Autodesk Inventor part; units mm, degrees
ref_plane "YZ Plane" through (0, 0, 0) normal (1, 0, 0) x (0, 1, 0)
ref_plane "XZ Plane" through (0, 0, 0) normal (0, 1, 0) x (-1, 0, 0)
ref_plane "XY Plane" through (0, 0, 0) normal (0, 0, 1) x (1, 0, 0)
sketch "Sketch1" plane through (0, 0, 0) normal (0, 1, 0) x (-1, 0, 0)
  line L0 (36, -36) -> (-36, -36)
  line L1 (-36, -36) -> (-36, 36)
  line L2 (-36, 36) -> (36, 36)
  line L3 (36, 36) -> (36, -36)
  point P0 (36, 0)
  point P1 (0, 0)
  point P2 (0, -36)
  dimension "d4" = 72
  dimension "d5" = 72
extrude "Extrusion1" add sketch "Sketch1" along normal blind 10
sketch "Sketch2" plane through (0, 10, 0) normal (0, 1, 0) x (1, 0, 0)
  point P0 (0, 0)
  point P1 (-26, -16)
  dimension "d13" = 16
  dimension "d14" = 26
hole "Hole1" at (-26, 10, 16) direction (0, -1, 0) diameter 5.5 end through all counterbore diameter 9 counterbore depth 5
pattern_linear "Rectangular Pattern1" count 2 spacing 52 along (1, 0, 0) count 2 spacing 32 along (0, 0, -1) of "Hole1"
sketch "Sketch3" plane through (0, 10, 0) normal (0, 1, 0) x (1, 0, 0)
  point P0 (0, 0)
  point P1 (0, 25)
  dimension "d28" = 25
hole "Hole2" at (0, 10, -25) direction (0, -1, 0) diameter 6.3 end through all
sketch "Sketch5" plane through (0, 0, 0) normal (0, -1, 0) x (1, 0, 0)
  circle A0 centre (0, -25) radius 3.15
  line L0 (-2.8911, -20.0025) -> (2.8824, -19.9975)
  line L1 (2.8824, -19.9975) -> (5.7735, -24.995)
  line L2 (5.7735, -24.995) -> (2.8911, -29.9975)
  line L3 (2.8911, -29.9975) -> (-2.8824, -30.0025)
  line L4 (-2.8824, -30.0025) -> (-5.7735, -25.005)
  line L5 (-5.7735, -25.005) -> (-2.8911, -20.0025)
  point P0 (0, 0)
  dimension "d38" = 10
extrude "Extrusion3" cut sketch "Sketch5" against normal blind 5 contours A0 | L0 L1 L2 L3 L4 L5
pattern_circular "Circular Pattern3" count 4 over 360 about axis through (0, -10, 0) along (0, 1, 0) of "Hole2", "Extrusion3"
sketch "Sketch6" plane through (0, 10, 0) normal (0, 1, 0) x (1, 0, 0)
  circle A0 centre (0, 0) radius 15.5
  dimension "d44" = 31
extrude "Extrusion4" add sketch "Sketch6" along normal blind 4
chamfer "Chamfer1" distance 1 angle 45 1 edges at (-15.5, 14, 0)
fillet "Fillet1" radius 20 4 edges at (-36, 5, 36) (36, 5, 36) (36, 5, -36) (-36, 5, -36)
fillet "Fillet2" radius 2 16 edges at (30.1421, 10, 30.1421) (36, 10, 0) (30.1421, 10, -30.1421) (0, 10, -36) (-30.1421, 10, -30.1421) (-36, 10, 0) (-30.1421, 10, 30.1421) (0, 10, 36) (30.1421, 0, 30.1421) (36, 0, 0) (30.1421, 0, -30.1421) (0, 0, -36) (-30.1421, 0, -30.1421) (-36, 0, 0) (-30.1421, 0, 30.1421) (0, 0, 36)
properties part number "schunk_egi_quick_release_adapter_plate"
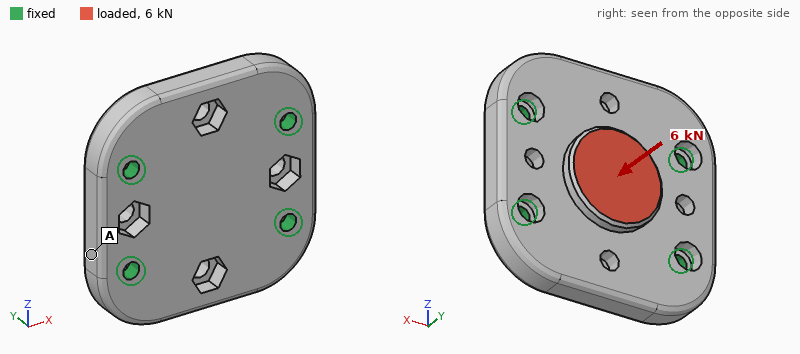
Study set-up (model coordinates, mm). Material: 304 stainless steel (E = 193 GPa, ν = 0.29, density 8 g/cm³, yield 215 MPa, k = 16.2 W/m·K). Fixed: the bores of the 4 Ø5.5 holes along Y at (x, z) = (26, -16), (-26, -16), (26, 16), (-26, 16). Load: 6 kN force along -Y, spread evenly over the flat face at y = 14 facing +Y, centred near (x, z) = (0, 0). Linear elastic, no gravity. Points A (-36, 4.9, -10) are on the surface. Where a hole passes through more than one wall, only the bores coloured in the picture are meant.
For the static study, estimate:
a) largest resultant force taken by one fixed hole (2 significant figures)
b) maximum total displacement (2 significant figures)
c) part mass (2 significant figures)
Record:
2.0 kN
7.6 µm
370 g
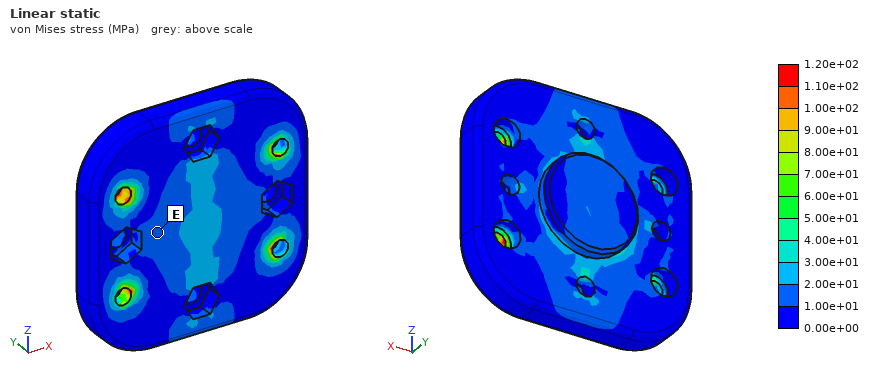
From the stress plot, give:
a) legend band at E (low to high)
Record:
1.00e+01 to 2.00e+01 MPa
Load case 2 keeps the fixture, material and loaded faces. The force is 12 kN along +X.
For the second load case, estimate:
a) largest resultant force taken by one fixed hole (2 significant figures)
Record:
3.5 kN
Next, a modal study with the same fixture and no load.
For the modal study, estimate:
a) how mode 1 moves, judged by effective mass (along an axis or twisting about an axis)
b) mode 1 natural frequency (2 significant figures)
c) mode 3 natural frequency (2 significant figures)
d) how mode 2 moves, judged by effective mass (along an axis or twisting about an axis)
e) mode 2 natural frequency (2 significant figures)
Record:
twisting about X
9500 Hz
15 kHz
along Y
9900 Hz
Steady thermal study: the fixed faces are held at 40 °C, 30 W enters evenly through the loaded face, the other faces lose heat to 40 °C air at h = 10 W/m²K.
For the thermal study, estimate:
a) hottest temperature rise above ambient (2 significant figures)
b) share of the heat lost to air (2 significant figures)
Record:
65 K
8.6 %
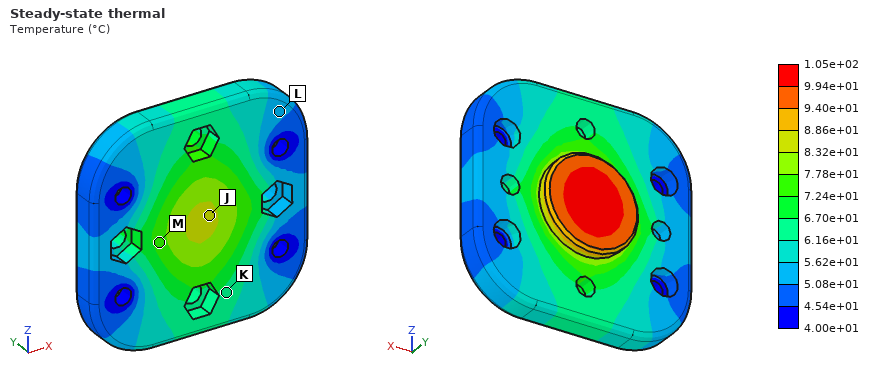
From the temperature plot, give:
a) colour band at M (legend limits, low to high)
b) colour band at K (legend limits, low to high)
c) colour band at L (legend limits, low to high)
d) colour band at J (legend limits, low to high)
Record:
7.24e+01 to 7.78e+01 °C
6.16e+01 to 6.70e+01 °C
5.08e+01 to 5.62e+01 °C
8.32e+01 to 8.86e+01 °C
